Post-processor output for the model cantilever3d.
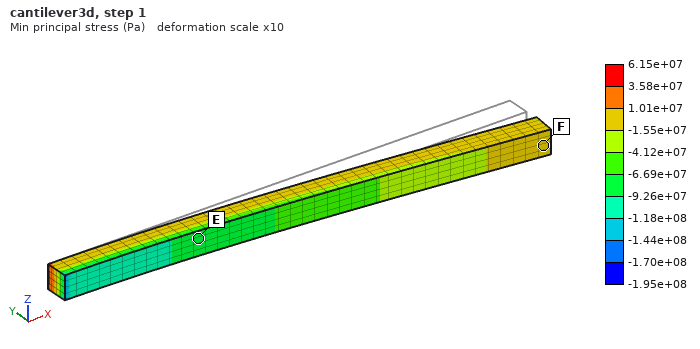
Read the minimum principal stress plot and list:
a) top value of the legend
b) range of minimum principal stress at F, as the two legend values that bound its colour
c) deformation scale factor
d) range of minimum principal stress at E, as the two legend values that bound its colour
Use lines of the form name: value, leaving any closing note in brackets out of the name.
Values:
top value of the legend: 6.15e+07 Pa
range of minimum principal stress at F, as the two legend values that bound its colour: -1.55e+07 to 1.01e+07 Pa
deformation scale factor: 10
range of minimum principal stress at E, as the two legend values that bound its colour: -9.26e+07 to -6.69e+07 Pa
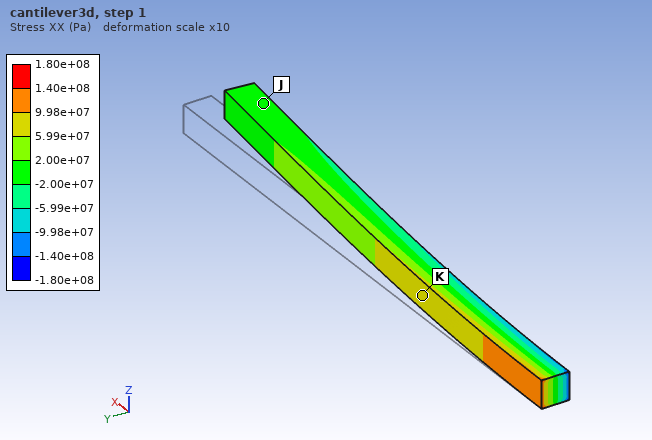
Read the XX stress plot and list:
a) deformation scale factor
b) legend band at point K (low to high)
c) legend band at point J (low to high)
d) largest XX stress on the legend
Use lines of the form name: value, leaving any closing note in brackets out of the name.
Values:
deformation scale factor: 10
legend band at point K: 5.99e+07 to 9.98e+07 Pa
legend band at point J: -2.00e+07 to 2.00e+07 Pa
largest XX stress on the legend: 1.80e+08 Pa
